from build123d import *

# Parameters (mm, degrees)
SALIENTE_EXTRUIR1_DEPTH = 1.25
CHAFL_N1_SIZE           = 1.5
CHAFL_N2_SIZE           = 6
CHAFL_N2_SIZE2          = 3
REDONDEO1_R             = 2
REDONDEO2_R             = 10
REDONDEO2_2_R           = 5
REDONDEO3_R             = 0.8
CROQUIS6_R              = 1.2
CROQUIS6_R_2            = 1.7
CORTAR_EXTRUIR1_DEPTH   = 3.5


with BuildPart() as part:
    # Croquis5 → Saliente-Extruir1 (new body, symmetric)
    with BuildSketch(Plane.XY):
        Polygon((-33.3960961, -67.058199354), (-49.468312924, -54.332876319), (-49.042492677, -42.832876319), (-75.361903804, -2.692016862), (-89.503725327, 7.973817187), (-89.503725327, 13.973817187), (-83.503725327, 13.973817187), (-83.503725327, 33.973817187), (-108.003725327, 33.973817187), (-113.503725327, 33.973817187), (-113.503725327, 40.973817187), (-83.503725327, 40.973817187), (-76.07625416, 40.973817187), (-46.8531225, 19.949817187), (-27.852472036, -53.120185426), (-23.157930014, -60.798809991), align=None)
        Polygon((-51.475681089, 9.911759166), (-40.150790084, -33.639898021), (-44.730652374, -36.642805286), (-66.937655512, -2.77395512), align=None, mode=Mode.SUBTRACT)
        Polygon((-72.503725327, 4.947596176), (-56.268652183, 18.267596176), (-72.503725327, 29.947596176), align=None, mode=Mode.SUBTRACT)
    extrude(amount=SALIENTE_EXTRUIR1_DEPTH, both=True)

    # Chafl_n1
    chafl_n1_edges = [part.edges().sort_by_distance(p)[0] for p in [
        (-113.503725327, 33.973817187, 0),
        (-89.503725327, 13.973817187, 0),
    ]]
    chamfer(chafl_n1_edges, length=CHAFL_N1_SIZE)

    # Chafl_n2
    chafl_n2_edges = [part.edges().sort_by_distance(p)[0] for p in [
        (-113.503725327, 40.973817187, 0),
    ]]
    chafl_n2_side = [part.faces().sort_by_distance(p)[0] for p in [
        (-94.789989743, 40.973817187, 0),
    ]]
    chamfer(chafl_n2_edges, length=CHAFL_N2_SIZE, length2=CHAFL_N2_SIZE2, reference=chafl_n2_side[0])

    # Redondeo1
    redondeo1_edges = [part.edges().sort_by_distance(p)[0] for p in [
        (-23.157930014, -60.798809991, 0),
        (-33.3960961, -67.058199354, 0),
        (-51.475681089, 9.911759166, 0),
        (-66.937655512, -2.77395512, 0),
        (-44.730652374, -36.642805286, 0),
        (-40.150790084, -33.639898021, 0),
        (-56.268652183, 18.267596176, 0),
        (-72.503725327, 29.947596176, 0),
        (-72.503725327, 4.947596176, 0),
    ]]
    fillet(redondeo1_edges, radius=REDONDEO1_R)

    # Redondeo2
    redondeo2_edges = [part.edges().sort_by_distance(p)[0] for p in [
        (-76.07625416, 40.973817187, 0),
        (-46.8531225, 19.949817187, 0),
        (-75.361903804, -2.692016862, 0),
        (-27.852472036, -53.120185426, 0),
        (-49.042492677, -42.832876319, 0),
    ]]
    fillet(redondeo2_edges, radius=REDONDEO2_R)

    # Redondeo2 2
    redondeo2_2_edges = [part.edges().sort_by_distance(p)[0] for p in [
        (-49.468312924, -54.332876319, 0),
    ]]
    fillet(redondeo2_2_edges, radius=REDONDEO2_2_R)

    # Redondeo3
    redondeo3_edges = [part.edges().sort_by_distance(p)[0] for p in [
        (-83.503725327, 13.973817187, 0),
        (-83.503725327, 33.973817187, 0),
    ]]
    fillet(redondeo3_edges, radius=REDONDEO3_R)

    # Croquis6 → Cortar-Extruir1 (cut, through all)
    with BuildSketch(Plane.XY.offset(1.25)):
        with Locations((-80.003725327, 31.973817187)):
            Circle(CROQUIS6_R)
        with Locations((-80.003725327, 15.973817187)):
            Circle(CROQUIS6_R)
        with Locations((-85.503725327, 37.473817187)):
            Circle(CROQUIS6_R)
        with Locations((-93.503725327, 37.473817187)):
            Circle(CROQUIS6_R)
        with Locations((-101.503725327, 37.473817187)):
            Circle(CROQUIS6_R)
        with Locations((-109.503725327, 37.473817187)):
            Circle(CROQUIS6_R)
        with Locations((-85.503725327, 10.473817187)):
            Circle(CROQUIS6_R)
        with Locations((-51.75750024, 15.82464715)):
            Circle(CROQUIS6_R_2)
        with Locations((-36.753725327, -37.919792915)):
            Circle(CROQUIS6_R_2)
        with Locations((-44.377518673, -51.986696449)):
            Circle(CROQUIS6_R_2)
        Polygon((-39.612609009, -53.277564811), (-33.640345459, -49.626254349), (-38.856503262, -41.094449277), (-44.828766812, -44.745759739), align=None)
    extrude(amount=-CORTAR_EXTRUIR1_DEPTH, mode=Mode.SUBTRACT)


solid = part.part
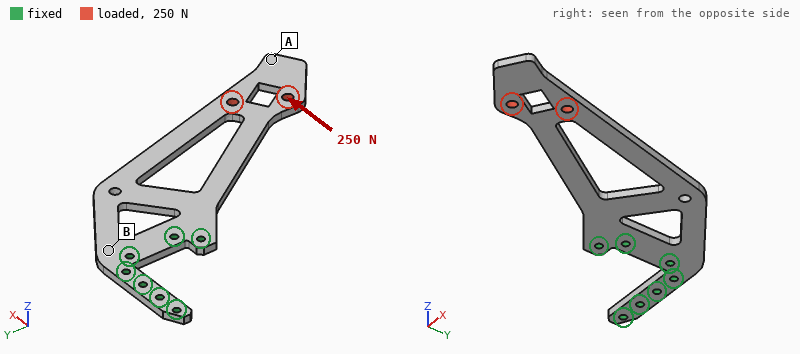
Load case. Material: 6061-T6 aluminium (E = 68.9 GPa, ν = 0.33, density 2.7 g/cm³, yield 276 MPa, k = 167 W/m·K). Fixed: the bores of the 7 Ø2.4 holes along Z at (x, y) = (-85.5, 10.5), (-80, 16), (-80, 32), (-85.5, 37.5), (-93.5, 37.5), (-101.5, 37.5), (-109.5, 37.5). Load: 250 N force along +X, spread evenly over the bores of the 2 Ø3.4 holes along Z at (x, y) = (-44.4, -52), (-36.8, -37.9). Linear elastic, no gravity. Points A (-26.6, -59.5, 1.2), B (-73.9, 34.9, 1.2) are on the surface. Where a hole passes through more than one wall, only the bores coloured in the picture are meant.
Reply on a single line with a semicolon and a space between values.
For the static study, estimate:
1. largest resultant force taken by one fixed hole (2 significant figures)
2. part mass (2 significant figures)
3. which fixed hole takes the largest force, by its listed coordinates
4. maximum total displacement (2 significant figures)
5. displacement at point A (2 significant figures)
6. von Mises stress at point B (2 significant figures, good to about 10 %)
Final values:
750 N; 15 g; (-85.5, 10.5); 0.21 mm; 0.20 mm; 21 MPa
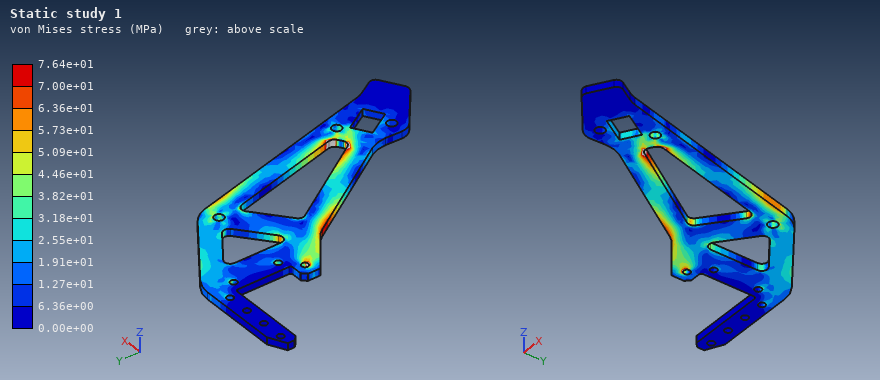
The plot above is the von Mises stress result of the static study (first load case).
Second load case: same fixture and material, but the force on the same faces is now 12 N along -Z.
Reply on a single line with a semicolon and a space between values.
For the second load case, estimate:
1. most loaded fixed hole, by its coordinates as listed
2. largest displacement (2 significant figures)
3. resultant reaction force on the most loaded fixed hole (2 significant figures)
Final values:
(-80, 16); 1.5 mm; 23 N
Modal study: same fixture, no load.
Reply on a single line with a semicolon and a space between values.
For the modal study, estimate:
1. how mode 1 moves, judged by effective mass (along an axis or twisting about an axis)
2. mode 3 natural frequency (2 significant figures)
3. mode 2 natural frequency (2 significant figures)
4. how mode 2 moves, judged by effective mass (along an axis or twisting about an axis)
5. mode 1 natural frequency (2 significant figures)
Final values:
along Z; 1800 Hz; 1100 Hz; along Z; 240 Hz
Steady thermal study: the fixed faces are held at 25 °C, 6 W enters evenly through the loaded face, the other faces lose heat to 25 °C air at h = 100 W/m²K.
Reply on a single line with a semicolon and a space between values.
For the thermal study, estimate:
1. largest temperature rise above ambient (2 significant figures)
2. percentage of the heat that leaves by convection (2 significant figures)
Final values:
26 K; 81 %
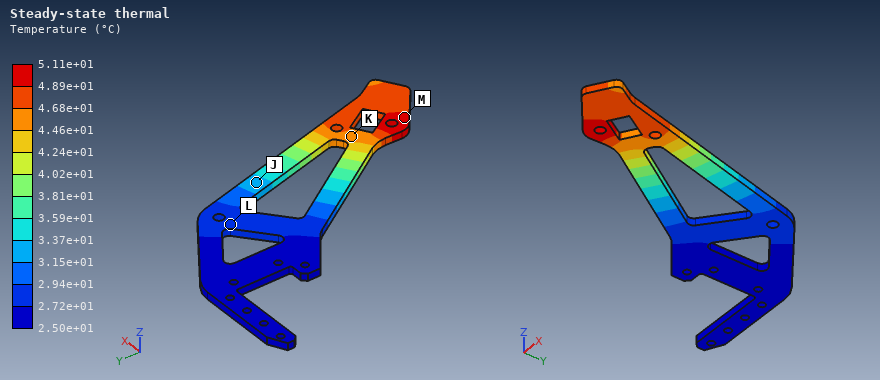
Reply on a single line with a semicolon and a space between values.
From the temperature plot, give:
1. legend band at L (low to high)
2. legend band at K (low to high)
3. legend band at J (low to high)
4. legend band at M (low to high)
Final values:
2.72e+01 to 2.94e+01 °C; 4.46e+01 to 4.68e+01 °C; 3.15e+01 to 3.37e+01 °C; 4.89e+01 to 5.11e+01 °C
